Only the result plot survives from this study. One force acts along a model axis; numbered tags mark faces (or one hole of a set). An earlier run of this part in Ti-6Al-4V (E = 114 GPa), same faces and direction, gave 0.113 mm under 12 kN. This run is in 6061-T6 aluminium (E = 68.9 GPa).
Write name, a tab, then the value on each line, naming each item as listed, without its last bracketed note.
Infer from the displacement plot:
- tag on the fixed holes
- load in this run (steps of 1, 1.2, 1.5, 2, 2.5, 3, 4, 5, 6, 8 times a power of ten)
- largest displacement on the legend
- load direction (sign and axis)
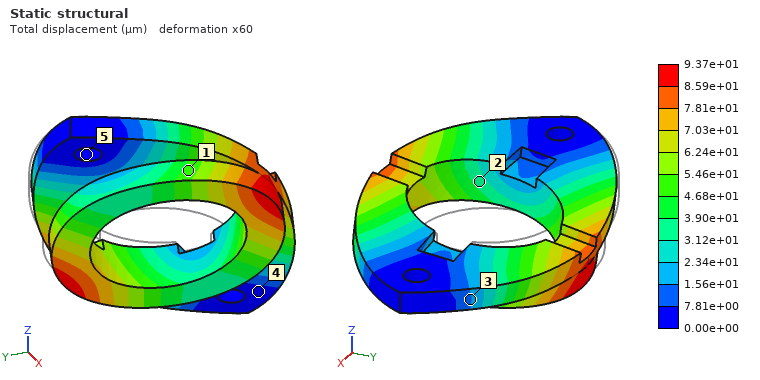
tag on the fixed holes	5
load in this run	6 kN
largest displacement on the legend	9.37e+01 µm
load direction	-Y
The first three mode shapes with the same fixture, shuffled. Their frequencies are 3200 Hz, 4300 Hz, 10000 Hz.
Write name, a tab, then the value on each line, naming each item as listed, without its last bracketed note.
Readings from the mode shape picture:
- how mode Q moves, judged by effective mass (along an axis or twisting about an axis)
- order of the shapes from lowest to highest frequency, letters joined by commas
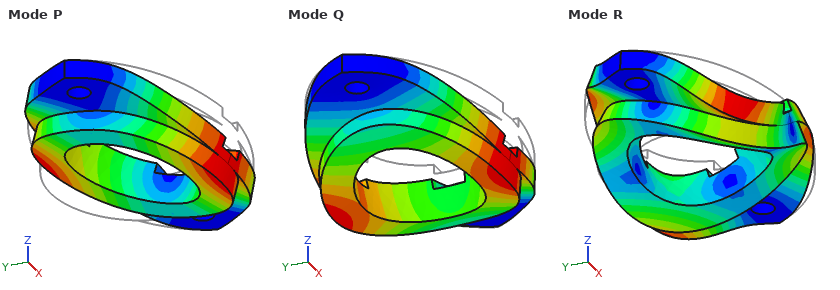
how mode Q moves, judged by effective mass	along Z
order of the shapes from lowest to highest frequency, letters joined by commas	P, Q, R
